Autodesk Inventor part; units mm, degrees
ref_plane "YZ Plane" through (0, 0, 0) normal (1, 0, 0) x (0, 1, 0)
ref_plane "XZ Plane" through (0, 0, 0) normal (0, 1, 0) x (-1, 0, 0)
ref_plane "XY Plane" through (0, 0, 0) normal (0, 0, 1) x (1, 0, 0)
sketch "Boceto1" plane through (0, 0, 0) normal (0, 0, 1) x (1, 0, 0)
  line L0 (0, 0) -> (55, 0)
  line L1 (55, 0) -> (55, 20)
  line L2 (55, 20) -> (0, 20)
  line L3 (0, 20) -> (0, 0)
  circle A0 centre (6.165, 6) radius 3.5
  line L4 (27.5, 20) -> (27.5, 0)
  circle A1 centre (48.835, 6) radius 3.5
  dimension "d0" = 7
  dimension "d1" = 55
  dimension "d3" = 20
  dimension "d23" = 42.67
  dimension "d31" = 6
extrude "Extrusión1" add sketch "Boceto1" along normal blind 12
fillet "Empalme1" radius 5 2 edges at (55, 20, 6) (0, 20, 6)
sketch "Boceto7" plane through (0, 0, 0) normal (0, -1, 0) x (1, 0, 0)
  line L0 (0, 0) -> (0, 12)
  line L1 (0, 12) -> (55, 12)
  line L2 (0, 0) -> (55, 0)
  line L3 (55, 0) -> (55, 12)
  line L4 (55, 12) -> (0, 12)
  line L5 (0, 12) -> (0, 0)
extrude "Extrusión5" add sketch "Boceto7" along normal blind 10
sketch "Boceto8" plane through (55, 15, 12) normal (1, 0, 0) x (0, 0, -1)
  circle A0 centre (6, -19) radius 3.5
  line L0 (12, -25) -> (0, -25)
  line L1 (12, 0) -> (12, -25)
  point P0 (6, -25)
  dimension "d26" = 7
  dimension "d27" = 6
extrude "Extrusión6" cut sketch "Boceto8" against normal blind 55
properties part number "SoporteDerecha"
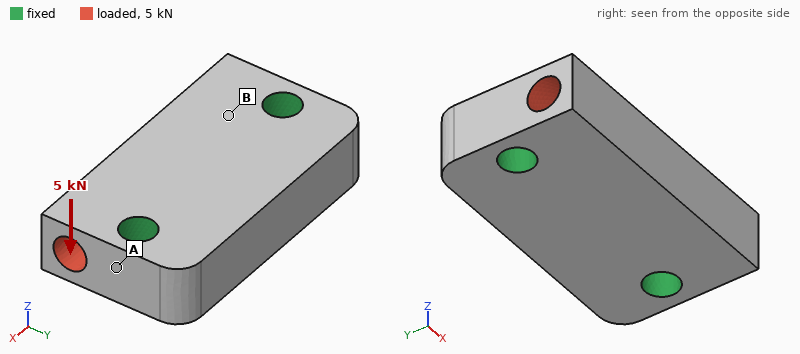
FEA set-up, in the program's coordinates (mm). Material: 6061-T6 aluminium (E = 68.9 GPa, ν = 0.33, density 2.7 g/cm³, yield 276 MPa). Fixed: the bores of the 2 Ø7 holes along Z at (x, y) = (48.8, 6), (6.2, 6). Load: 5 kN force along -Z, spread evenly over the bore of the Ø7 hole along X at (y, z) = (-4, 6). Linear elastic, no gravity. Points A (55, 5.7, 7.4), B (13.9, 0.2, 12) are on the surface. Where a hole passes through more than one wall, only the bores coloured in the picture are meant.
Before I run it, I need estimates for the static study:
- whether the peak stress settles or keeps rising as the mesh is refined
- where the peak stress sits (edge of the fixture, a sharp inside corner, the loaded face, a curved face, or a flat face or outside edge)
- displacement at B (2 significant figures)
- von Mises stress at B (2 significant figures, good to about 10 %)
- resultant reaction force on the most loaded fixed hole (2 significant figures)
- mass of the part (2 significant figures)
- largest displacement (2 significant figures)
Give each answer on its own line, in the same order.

keeps rising
edge of the fixture
8.8 µm
33 MPa
2.5 kN
45 g
28 µm
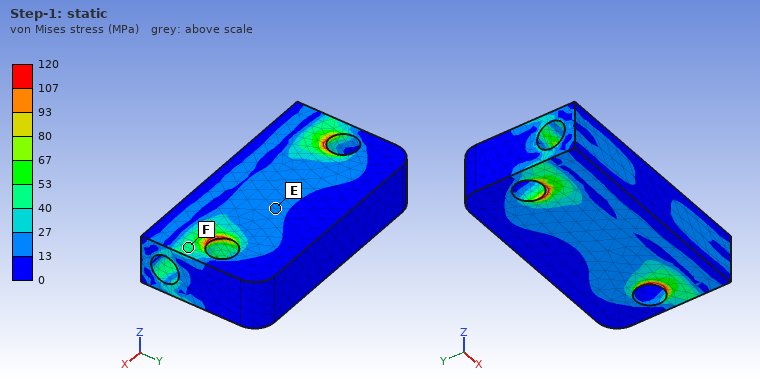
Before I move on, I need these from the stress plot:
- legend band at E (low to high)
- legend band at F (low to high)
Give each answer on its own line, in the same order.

13 to 27 MPa
40 to 53 MPa
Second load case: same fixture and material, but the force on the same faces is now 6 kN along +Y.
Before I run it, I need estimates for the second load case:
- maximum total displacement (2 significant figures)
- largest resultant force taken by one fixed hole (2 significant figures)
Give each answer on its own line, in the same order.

7.4 µm
3.0 kN
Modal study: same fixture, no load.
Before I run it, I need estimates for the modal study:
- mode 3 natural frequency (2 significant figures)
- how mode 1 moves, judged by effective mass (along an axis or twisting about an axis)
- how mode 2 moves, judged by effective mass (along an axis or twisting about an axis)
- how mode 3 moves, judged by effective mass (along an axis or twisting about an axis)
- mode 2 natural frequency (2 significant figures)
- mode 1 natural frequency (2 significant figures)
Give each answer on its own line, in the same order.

28 kHz
along Z
along Z
along Y
23 kHz
20 kHz
